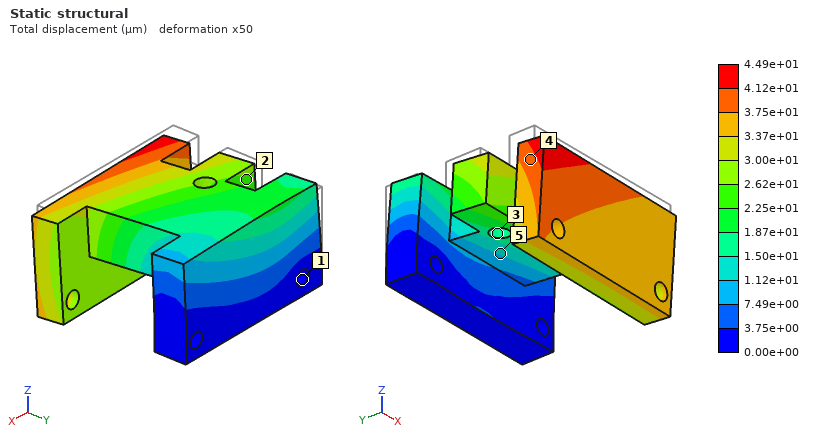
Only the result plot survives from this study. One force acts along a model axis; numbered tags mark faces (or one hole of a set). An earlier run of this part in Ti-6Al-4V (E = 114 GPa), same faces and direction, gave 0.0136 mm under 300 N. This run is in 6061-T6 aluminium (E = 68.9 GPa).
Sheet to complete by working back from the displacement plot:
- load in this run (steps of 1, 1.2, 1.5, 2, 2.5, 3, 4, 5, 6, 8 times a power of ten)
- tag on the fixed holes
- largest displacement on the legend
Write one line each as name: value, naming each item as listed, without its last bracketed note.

load in this run: 600 N
tag on the fixed holes: 1
largest displacement on the legend: 4.49e+01 µm
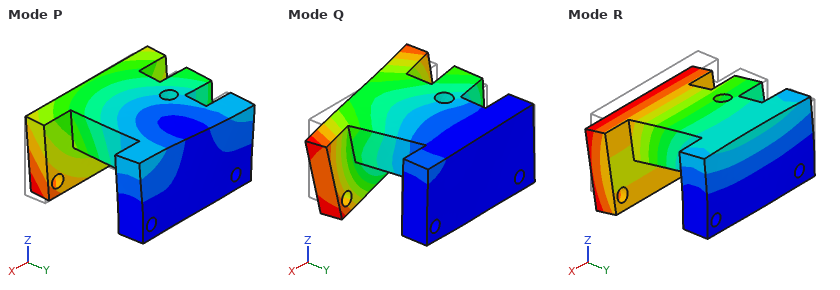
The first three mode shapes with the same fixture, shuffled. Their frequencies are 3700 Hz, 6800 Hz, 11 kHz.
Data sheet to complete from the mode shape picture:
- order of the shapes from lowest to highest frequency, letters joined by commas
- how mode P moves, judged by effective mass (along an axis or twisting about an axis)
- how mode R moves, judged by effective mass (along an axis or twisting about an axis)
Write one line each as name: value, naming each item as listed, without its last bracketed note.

order of the shapes from lowest to highest frequency, letters joined by commas: R, P, Q
how mode P moves, judged by effective mass: along X
how mode R moves, judged by effective mass: along Z
